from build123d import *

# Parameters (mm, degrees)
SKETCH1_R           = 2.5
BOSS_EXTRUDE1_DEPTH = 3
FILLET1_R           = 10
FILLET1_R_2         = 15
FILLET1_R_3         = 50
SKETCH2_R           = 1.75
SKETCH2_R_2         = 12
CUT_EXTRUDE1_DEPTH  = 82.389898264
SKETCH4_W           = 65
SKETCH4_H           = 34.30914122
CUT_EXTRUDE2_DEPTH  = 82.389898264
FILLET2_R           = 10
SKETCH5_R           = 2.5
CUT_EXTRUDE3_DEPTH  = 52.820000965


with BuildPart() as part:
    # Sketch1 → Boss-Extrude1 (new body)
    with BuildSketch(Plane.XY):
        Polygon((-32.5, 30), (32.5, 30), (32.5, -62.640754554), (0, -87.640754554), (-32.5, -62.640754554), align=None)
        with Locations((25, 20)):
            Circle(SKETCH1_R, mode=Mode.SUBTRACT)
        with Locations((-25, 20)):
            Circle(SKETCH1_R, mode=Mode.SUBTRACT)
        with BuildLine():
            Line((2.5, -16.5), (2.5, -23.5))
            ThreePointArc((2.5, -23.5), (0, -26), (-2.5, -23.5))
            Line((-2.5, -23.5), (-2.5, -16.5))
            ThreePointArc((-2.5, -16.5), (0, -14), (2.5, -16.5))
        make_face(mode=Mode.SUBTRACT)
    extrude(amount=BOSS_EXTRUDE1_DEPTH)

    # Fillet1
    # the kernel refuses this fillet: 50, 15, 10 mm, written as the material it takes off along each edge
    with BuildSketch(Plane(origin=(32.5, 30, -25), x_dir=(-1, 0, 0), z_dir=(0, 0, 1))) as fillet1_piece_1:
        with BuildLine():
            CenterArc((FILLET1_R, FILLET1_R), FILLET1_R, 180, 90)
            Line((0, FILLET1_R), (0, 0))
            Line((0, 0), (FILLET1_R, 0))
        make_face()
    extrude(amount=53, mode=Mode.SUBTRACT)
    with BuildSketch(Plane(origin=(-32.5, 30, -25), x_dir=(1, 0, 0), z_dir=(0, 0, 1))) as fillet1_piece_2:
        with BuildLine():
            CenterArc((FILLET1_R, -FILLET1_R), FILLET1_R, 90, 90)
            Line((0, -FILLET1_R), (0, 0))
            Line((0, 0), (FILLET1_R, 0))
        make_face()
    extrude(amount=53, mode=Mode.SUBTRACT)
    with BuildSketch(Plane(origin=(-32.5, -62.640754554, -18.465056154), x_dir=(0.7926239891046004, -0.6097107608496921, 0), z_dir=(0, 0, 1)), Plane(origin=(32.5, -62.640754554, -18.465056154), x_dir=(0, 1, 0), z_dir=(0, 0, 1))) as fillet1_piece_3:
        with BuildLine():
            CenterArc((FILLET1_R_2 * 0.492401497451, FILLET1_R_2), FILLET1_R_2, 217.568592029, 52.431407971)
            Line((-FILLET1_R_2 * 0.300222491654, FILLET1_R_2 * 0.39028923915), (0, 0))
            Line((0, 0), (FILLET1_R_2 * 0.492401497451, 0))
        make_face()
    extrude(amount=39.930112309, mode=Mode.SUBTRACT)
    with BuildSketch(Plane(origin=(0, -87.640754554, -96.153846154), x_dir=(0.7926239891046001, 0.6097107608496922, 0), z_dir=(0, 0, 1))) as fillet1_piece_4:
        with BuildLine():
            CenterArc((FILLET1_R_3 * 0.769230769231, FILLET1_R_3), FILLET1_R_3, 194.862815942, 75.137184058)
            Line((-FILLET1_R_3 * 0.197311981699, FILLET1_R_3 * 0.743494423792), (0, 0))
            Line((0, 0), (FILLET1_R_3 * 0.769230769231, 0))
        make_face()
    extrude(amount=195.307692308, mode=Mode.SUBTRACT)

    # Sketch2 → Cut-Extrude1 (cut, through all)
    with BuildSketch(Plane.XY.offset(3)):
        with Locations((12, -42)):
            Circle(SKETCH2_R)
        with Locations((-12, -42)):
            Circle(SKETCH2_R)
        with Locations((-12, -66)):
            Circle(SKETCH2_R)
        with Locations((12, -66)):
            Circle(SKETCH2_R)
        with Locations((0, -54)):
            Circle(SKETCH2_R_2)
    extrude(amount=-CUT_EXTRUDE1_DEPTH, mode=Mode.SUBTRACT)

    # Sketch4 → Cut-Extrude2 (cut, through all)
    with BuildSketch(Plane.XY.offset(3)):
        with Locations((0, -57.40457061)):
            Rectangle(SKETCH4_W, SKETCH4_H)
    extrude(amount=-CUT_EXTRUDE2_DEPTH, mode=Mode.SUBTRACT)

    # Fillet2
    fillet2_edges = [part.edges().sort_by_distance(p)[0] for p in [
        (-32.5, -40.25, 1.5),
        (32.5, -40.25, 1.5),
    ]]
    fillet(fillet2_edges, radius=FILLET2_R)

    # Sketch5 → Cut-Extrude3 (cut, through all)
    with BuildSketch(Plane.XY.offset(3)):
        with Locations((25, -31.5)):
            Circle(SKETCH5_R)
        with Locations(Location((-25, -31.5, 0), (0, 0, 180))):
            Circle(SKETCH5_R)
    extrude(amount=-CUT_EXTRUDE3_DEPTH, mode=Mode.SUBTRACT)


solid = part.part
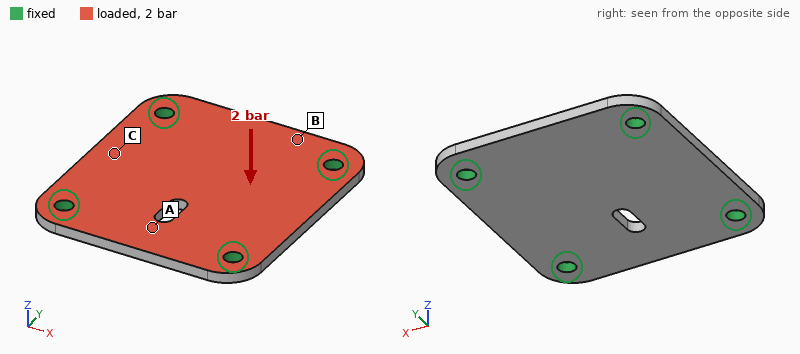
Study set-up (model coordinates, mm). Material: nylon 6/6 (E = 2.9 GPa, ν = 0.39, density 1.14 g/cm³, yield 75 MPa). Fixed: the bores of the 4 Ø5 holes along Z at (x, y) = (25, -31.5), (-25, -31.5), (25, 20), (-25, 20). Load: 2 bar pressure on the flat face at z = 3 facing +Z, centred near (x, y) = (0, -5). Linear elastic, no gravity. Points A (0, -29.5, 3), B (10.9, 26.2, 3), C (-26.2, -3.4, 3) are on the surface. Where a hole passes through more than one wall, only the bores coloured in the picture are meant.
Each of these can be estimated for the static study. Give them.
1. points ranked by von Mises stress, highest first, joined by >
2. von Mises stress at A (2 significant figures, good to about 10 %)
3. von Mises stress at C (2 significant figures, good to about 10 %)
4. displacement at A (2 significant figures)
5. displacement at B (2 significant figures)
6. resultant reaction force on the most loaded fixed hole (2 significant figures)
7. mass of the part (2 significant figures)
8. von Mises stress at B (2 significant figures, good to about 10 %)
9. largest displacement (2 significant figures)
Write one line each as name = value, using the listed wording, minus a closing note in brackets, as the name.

points ranked by von Mises stress, highest first, joined by > = A > C > B
von Mises stress at A = 19 MPa
von Mises stress at C = 15 MPa
displacement at A = 0.64 mm
displacement at B = 0.29 mm
resultant reaction force on the most loaded fixed hole = 220 N
mass of the part = 15 g
von Mises stress at B = 5.6 MPa
largest displacement = 1.1 mm
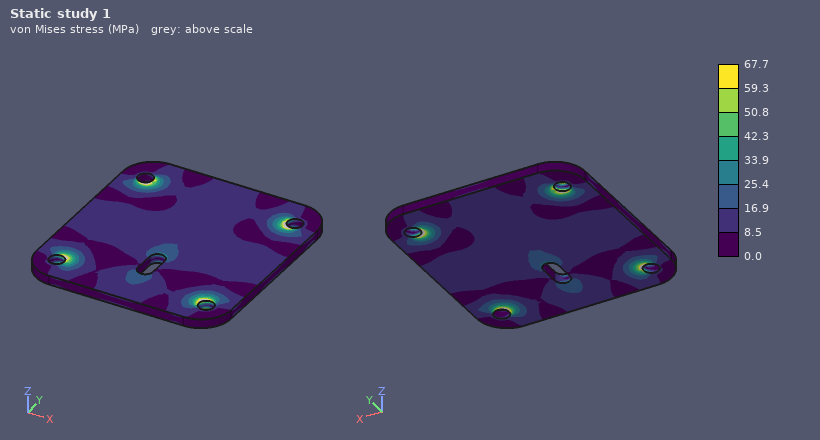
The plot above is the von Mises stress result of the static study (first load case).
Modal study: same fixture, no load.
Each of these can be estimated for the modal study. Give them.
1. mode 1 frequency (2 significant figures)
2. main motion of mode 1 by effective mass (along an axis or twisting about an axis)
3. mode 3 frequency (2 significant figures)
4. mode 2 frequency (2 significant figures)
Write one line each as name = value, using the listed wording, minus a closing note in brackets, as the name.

mode 1 frequency = 1400 Hz
main motion of mode 1 by effective mass = along Z
mode 3 frequency = 2200 Hz
mode 2 frequency = 2200 Hz
